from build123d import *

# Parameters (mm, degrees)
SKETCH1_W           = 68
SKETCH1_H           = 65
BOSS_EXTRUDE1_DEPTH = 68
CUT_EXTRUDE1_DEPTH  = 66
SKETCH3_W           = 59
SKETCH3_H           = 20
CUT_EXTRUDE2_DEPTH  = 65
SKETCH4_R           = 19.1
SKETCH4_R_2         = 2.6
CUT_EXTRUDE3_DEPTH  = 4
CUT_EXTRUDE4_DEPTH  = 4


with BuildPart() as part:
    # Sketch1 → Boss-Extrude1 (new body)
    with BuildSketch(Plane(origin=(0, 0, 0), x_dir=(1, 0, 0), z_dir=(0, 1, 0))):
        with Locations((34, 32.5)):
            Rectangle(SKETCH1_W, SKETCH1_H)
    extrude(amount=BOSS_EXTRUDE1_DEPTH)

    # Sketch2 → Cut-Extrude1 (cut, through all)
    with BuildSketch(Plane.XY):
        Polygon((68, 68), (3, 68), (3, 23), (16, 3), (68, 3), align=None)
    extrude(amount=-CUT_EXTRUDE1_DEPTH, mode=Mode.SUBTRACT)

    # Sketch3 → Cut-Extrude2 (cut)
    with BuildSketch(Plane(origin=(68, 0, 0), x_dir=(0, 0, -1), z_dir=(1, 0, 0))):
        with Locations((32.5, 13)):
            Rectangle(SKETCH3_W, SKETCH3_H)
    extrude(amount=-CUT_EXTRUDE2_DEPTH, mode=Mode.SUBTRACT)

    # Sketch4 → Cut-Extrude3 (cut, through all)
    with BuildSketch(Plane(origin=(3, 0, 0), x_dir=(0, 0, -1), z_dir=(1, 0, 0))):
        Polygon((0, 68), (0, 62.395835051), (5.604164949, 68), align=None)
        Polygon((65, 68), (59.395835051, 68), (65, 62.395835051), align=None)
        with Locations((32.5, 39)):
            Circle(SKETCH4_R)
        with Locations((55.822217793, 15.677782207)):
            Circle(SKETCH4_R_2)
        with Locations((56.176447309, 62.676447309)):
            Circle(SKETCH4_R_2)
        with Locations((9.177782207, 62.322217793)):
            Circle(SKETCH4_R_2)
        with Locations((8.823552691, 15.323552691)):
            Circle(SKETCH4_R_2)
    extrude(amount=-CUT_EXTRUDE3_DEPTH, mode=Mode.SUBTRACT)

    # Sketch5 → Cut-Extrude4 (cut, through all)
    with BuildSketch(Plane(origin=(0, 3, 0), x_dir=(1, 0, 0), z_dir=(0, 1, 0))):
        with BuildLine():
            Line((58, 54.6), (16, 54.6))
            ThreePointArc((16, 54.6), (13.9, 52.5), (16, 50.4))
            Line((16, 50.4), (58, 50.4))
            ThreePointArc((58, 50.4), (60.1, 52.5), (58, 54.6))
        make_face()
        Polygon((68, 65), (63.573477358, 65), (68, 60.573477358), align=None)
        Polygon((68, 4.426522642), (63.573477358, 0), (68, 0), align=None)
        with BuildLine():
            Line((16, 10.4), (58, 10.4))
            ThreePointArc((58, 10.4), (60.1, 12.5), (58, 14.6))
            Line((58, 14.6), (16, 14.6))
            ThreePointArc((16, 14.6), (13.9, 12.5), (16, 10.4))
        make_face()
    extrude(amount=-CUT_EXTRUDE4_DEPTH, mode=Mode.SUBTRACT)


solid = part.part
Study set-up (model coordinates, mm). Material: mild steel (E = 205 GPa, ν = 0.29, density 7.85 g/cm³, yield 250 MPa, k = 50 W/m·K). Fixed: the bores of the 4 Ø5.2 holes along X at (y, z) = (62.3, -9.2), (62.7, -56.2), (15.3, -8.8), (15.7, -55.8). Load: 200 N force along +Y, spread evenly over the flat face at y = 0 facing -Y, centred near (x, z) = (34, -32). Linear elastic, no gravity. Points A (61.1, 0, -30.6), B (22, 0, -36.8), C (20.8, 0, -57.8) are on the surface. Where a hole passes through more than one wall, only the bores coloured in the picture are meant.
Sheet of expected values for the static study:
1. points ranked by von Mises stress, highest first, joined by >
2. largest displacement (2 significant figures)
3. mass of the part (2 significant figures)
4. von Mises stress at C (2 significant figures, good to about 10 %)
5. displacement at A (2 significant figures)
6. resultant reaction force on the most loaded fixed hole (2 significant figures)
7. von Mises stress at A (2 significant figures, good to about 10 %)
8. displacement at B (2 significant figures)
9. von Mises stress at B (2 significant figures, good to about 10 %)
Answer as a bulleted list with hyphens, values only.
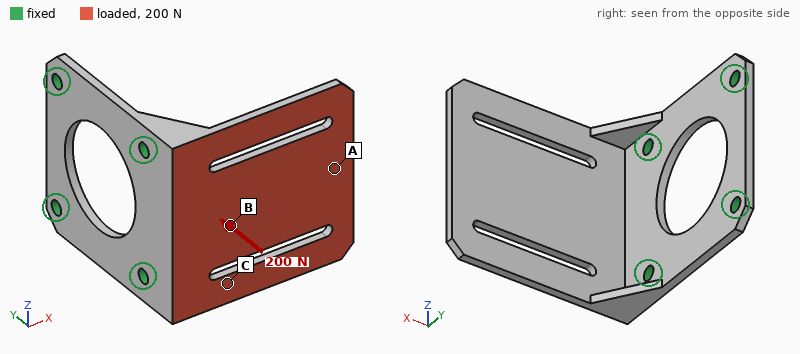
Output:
- C > B > A
- 0.27 mm
- 170 g
- 51 MPa
- 0.23 mm
- 110 N
- 7.5 MPa
- 0.054 mm
- 26 MPa
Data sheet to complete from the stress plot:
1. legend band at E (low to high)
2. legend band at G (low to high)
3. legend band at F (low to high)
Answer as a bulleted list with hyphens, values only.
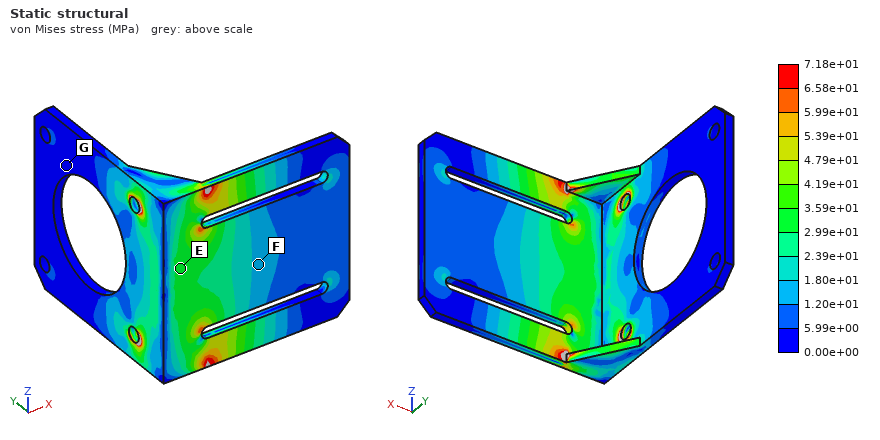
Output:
- 2.99e+01 to 3.59e+01 MPa
- 0.00e+00 to 5.99e+00 MPa
- 1.20e+01 to 1.80e+01 MPa
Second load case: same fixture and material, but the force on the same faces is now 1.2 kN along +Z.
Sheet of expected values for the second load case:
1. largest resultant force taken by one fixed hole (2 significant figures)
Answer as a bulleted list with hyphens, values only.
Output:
- 1.0 kN
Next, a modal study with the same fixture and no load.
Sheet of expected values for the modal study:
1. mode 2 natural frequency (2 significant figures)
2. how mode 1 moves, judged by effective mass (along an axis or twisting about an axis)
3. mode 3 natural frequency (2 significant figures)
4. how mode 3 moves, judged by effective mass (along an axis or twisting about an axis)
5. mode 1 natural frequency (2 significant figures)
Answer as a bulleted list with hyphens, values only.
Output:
- 1500 Hz
- along Y
- 2300 Hz
- along Z
- 560 Hz
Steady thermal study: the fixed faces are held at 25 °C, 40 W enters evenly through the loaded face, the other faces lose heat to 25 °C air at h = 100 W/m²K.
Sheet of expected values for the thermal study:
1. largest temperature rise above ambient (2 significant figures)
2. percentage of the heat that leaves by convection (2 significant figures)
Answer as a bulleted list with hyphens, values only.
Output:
- 61 K
- 70 %
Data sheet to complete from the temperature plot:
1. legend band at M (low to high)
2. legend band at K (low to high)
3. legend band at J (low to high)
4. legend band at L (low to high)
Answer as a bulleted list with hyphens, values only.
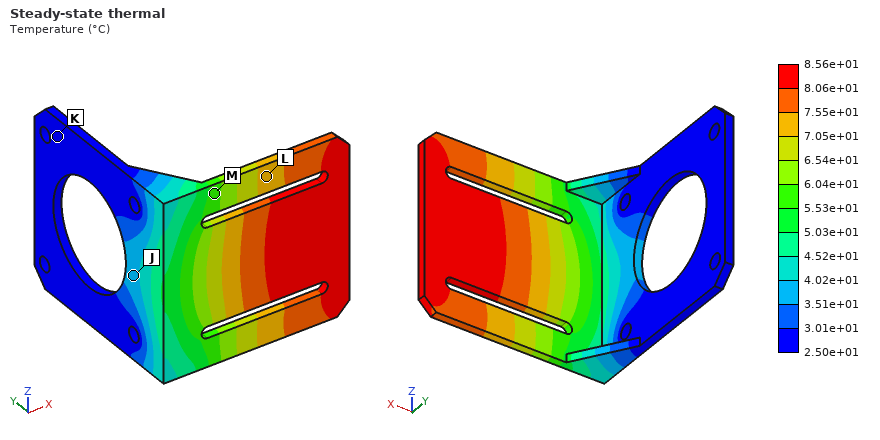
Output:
- 5.53e+01 to 6.04e+01 °C
- 2.50e+01 to 3.01e+01 °C
- 3.51e+01 to 4.02e+01 °C
- 7.05e+01 to 7.55e+01 °C
